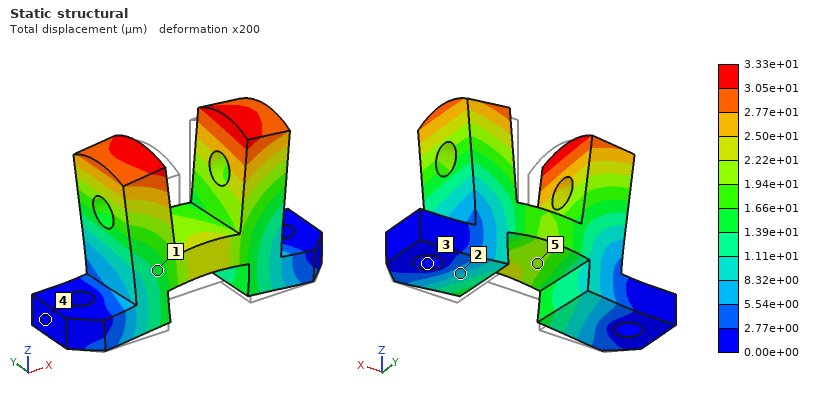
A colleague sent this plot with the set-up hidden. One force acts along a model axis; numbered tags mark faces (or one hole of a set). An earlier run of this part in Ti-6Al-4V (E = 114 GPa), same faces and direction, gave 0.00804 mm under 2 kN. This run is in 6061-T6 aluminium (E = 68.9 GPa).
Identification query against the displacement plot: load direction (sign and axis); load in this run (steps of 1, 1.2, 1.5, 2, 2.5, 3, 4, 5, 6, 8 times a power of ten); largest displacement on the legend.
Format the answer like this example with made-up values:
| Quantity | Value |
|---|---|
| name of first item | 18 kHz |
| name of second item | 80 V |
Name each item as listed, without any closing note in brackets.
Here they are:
| Quantity | Value |
|---|---|
| load direction | +Z |
| load in this run | 5 kN |
| largest displacement on the legend | 3.33e+01 µm |
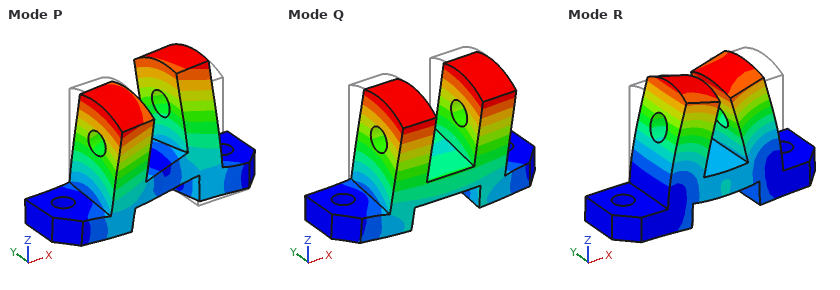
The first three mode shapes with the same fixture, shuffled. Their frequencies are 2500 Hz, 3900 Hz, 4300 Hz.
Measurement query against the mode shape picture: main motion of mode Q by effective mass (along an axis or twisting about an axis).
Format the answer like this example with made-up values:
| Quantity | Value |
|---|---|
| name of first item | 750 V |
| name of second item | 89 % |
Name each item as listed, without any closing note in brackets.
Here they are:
| Quantity | Value |
|---|---|
| main motion of mode Q by effective mass | along Y |
